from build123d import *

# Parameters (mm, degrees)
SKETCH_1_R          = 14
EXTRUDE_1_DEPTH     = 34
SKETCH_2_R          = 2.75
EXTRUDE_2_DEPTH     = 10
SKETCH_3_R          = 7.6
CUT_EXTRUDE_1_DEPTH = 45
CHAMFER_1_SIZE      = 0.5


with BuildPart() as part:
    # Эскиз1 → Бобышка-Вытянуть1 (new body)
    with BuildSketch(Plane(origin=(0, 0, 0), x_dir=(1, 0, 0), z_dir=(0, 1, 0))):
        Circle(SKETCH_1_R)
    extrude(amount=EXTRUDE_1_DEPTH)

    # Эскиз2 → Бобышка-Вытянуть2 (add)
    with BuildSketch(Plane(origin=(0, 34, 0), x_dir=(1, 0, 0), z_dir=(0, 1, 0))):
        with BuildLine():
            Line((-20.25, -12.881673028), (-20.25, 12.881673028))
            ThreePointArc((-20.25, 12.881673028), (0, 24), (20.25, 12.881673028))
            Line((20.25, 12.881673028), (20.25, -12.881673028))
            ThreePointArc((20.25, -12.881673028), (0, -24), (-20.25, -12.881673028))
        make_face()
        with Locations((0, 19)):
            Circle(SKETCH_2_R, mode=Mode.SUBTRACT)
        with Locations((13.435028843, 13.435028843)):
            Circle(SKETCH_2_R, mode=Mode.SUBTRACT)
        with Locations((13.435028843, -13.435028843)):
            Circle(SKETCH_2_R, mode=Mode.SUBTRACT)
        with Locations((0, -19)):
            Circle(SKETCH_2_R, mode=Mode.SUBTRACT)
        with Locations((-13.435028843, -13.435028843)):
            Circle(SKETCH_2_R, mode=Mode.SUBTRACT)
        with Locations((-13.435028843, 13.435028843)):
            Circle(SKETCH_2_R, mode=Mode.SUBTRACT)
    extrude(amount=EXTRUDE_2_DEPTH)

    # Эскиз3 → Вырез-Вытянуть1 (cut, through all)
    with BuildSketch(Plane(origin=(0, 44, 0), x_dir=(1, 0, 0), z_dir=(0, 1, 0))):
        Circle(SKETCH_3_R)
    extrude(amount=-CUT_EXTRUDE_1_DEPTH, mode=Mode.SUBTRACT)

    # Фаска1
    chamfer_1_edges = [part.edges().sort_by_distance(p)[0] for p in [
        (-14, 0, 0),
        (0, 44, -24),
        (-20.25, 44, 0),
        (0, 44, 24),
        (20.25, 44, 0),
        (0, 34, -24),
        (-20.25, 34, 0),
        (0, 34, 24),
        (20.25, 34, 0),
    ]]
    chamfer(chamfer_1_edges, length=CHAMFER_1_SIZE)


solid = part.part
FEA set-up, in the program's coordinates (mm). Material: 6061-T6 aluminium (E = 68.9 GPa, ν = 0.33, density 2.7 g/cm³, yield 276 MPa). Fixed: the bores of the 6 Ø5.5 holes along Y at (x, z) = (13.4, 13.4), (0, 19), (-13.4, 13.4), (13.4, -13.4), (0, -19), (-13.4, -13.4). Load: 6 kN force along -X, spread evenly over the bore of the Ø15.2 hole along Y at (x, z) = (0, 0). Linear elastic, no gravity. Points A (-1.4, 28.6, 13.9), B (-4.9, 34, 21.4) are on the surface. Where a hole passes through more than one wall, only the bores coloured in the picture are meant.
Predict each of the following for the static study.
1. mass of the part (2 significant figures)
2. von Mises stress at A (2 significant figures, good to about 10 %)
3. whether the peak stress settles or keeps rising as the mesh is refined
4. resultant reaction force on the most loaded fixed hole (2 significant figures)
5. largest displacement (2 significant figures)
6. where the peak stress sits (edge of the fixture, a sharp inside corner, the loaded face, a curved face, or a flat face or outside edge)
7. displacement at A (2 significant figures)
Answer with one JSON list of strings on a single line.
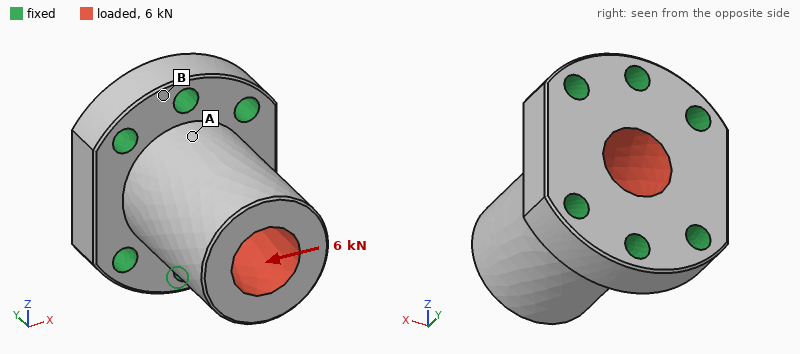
["76 g", "19 MPa", "keeps rising", "2.3 kN", "41 µm", "edge of the fixture", "7.6 µm"]
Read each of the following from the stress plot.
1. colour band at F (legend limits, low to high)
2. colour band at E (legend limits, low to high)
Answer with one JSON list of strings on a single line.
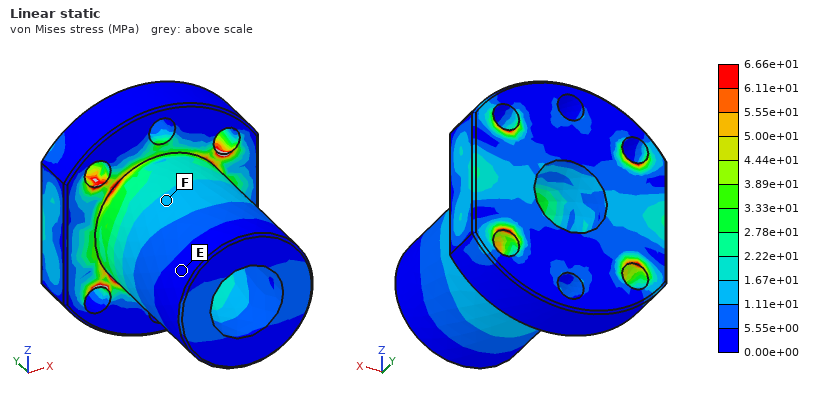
["1.11e+01 to 1.67e+01 MPa", "0.00e+00 to 5.55e+00 MPa"]
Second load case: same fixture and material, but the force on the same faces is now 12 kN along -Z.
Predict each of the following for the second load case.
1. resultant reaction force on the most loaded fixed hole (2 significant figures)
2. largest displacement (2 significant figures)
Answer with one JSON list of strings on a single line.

["4.0 kN", "70 µm"]
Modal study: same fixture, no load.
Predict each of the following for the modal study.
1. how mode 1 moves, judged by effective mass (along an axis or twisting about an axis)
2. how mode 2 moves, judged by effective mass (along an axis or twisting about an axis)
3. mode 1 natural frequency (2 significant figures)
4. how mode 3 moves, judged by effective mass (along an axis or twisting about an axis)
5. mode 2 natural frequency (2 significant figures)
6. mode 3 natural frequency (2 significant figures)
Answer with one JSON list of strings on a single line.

["along X", "along Z", "10 kHz", "twisting about Y", "11 kHz", "21 kHz"]
